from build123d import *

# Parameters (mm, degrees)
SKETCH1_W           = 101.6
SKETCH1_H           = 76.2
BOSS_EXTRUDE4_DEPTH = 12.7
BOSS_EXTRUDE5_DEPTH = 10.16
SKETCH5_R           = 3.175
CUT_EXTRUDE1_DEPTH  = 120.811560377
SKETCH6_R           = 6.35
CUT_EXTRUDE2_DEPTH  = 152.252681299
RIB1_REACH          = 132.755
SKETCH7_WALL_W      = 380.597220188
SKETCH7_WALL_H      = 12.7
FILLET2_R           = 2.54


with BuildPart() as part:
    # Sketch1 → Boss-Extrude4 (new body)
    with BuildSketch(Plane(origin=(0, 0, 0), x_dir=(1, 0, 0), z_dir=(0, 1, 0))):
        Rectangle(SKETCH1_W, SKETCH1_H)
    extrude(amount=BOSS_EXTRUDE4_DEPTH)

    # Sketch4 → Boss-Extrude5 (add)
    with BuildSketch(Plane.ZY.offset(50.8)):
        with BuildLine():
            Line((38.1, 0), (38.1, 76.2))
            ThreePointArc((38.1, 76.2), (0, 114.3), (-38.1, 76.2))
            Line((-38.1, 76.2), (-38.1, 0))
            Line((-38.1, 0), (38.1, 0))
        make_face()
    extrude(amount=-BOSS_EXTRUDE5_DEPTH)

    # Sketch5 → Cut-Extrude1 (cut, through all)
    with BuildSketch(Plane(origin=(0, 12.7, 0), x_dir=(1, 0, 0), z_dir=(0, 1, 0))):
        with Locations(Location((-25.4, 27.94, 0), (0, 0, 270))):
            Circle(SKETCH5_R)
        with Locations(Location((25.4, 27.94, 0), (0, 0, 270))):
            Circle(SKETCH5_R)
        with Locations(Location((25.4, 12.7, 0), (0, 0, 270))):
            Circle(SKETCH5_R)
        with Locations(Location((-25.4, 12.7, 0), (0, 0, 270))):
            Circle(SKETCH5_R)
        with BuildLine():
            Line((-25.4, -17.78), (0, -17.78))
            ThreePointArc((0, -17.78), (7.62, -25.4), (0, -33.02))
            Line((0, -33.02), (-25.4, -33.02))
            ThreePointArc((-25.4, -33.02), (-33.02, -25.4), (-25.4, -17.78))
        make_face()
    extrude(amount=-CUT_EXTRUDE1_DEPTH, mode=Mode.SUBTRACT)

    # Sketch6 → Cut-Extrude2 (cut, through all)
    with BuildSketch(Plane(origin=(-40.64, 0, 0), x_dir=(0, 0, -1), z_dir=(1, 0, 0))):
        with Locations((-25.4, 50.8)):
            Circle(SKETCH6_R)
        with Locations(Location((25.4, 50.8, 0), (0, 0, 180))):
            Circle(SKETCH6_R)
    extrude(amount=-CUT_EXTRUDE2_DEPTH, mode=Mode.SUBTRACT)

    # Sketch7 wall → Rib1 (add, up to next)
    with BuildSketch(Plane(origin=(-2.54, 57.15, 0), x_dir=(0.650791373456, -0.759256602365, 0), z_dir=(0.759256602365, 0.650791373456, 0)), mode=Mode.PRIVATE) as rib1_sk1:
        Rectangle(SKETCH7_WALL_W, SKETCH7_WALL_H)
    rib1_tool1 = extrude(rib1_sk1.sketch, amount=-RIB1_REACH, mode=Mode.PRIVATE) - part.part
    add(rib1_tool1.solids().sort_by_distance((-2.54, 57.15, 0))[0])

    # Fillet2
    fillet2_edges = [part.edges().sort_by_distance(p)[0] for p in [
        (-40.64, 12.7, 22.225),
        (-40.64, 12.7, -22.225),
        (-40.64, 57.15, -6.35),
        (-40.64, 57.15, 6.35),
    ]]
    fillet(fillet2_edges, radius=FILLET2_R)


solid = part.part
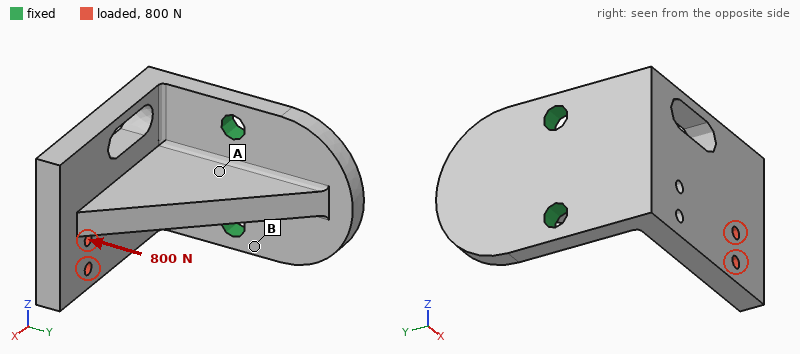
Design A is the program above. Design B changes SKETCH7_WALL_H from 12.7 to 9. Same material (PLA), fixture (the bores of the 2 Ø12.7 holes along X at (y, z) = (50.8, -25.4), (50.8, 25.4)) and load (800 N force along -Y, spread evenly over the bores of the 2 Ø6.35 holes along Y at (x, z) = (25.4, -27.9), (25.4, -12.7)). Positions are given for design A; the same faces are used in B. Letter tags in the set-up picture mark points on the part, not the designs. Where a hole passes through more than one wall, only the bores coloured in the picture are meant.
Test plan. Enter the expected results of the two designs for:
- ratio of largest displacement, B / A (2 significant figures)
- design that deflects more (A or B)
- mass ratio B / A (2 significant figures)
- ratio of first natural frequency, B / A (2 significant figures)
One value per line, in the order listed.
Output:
1.1
B
0.94
0.99
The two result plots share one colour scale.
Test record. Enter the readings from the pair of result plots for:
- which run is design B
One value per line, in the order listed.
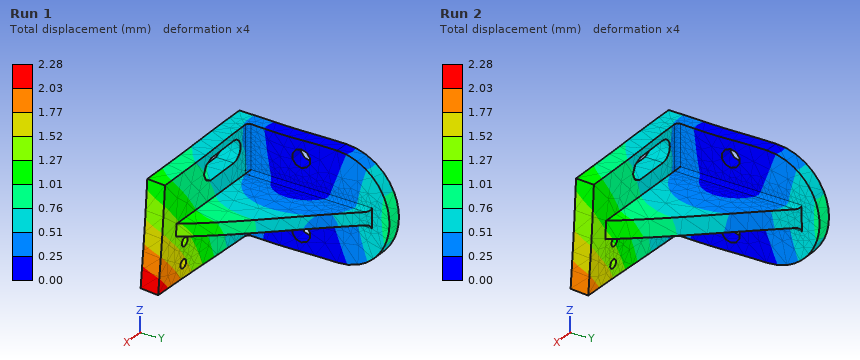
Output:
Run 1
